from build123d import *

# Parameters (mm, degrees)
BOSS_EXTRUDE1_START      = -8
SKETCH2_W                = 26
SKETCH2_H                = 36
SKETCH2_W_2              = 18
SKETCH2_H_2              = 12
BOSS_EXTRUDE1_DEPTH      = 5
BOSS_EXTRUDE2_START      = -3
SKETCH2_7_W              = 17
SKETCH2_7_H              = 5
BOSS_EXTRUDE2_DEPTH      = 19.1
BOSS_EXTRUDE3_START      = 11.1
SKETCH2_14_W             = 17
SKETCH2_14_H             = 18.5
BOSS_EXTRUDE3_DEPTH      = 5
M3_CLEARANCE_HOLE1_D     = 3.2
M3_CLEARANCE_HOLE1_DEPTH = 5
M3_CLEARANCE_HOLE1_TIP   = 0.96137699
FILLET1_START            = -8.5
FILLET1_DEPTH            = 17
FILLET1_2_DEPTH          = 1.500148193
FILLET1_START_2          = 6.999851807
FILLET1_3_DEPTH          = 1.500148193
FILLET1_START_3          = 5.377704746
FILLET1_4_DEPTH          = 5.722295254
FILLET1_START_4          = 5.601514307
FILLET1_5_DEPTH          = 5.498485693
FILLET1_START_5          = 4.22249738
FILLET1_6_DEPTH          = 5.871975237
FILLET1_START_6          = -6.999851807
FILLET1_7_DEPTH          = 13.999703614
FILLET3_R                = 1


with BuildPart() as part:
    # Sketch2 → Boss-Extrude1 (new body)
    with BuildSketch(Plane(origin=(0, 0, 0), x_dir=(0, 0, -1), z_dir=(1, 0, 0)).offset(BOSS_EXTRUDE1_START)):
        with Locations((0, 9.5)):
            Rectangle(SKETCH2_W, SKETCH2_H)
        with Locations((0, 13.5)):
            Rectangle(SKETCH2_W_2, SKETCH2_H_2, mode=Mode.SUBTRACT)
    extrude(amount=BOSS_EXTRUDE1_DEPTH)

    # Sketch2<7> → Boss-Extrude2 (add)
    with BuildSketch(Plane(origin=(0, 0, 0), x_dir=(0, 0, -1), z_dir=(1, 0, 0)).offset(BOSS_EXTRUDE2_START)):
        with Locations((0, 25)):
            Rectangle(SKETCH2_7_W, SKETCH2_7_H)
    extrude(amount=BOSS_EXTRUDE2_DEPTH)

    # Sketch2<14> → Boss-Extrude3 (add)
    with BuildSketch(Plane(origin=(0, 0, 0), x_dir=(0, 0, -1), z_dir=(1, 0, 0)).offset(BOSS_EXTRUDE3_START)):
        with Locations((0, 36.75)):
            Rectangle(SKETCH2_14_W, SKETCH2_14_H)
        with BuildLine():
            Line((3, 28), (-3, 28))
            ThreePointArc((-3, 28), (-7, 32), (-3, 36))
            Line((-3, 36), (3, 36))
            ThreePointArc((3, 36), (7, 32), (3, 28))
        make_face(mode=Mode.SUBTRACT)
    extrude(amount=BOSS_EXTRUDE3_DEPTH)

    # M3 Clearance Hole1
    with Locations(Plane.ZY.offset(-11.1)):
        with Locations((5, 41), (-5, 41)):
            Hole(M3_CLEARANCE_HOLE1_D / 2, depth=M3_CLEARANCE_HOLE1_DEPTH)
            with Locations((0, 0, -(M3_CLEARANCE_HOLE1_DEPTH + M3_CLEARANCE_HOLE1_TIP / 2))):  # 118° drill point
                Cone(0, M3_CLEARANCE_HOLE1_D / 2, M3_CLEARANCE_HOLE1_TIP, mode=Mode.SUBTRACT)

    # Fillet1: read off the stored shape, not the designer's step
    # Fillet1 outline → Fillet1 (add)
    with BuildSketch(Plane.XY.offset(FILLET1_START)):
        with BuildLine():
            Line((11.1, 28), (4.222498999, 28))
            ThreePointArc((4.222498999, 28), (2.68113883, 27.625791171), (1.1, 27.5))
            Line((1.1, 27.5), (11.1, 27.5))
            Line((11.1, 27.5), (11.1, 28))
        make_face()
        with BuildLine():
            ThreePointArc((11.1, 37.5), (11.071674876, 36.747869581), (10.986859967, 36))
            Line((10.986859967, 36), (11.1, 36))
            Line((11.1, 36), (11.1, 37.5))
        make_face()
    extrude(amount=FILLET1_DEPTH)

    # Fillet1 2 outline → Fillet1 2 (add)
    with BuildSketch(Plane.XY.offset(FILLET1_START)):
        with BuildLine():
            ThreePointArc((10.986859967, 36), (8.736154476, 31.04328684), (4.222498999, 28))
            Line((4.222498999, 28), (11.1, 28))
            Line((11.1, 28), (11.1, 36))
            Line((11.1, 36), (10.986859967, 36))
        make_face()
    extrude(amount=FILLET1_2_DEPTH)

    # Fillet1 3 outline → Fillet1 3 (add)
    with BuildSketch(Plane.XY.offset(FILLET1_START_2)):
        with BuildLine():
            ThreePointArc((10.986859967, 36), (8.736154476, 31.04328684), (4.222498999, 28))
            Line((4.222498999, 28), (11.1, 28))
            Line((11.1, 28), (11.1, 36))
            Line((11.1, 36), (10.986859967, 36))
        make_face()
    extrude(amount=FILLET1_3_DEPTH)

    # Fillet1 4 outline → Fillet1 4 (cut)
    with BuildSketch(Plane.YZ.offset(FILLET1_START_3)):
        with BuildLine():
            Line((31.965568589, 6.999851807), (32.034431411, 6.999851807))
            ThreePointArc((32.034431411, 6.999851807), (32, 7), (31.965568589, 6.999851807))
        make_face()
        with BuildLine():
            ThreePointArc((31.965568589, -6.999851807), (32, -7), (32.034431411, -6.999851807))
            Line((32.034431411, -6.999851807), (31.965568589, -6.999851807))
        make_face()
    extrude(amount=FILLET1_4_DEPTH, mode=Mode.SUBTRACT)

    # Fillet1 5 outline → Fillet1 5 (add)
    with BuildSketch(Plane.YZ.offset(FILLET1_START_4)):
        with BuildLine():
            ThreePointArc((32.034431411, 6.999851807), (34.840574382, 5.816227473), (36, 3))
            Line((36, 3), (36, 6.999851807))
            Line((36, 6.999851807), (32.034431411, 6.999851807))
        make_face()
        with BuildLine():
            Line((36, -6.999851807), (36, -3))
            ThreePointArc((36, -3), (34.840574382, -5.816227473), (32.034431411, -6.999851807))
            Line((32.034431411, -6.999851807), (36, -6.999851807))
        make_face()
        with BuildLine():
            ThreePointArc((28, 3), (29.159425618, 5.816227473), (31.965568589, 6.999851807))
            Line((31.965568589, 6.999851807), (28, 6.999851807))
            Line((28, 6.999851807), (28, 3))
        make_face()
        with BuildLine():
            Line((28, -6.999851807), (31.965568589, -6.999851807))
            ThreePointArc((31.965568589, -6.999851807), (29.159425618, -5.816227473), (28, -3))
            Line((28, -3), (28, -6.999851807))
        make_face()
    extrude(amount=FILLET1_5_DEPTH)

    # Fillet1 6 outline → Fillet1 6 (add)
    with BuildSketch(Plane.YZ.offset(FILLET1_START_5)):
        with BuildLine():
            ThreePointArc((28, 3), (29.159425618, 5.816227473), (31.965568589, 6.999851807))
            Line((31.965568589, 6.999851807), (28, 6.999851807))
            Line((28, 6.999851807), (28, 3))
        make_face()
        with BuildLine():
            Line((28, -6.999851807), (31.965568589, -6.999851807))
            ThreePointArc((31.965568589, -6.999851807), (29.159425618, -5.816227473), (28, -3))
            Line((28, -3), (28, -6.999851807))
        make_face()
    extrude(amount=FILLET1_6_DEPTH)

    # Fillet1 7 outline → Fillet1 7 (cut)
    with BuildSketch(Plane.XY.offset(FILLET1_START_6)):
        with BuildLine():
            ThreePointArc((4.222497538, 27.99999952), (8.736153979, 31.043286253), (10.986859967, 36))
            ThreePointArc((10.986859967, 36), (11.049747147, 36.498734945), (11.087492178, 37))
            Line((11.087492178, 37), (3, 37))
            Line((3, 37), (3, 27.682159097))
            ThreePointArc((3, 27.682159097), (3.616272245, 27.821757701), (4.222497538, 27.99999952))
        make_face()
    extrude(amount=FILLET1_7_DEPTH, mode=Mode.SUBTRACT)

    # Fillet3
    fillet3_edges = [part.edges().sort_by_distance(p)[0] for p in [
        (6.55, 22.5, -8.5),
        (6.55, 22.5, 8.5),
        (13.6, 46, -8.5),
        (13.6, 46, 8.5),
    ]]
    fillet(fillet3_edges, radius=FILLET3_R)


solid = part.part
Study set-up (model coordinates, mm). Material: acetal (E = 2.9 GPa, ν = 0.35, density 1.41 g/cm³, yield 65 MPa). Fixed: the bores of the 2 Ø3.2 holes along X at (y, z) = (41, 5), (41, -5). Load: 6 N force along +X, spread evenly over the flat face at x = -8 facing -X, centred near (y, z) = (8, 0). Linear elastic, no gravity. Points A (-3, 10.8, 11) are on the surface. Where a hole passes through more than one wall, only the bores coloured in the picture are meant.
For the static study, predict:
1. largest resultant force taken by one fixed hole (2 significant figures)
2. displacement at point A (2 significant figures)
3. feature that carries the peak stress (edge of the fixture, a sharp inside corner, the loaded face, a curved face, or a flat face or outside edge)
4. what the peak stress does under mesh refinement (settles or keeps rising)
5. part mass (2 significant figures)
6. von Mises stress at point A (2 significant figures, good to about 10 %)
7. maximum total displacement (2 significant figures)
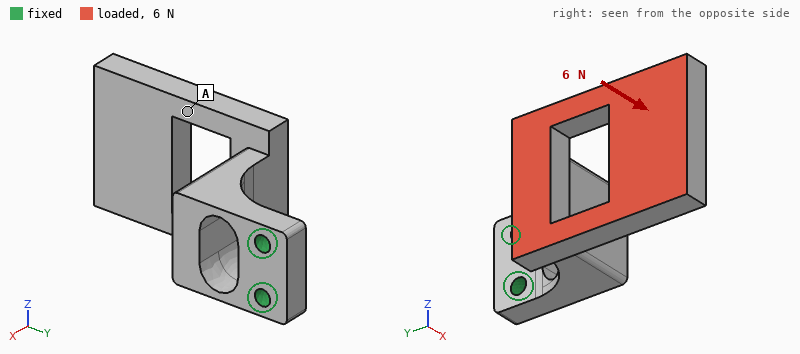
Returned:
3.0 N
0.33 mm
a sharp inside corner
keeps rising
9.0 g
1.2 MPa
0.64 mm
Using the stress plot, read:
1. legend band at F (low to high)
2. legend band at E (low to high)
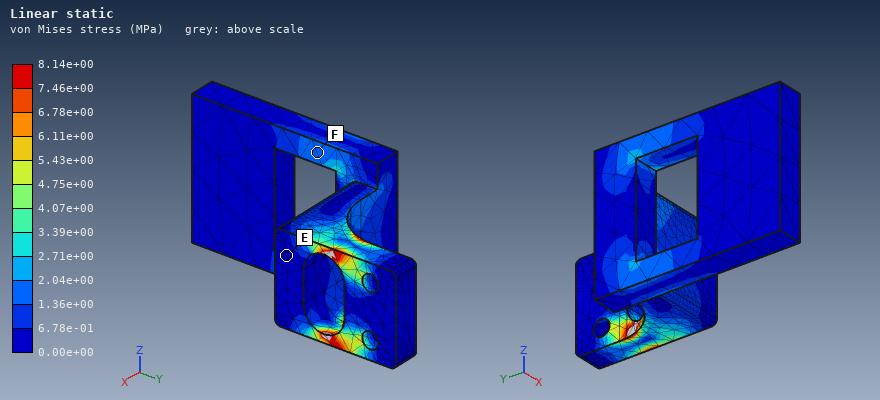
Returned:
1.36e+00 to 2.04e+00 MPa
0.00e+00 to 6.78e-01 MPa
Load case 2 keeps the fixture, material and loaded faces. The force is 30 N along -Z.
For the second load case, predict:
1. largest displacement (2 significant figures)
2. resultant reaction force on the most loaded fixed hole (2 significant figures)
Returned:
0.63 mm
87 N
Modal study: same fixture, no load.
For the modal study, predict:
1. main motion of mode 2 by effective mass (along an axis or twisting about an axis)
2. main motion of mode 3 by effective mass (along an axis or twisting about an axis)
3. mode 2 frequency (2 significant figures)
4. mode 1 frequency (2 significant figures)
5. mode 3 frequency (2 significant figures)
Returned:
along Z
along Y
550 Hz
230 Hz
920 Hz
